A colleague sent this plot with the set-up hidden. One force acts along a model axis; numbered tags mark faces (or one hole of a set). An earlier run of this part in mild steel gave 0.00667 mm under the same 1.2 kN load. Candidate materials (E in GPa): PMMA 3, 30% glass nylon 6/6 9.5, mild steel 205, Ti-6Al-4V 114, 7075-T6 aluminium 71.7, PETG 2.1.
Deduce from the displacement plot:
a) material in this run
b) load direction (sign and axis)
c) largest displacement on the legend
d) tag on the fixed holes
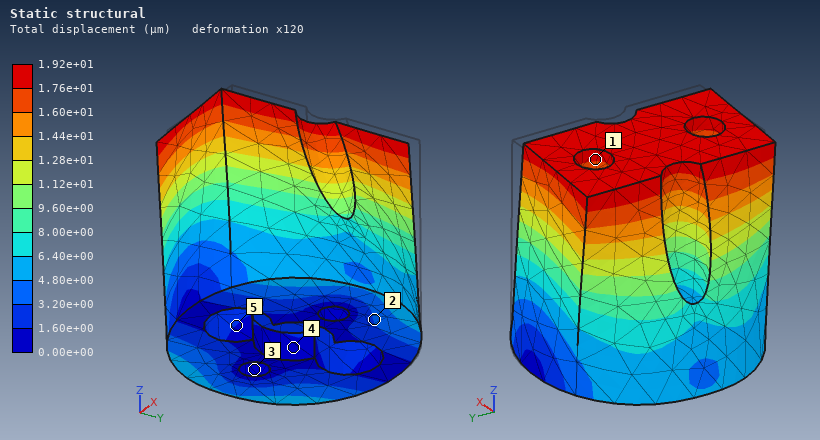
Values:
7075-T6 aluminium
-X
1.92e+01 µm
3
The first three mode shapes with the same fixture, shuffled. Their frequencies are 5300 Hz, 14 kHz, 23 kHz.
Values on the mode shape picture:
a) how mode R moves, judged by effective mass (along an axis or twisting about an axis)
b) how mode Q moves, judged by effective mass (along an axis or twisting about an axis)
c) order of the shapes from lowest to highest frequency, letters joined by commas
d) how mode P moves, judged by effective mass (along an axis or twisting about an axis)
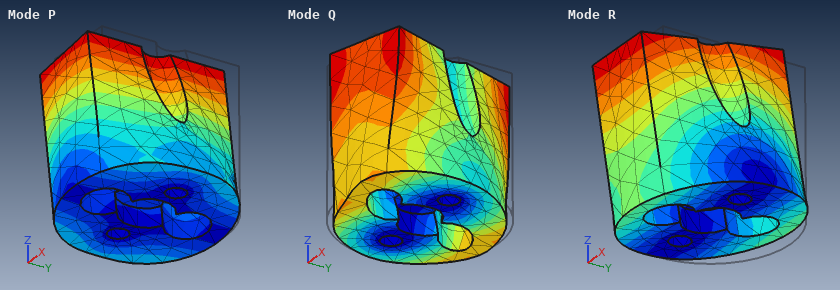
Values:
along Y
twisting about Z
R, P, Q
along X
